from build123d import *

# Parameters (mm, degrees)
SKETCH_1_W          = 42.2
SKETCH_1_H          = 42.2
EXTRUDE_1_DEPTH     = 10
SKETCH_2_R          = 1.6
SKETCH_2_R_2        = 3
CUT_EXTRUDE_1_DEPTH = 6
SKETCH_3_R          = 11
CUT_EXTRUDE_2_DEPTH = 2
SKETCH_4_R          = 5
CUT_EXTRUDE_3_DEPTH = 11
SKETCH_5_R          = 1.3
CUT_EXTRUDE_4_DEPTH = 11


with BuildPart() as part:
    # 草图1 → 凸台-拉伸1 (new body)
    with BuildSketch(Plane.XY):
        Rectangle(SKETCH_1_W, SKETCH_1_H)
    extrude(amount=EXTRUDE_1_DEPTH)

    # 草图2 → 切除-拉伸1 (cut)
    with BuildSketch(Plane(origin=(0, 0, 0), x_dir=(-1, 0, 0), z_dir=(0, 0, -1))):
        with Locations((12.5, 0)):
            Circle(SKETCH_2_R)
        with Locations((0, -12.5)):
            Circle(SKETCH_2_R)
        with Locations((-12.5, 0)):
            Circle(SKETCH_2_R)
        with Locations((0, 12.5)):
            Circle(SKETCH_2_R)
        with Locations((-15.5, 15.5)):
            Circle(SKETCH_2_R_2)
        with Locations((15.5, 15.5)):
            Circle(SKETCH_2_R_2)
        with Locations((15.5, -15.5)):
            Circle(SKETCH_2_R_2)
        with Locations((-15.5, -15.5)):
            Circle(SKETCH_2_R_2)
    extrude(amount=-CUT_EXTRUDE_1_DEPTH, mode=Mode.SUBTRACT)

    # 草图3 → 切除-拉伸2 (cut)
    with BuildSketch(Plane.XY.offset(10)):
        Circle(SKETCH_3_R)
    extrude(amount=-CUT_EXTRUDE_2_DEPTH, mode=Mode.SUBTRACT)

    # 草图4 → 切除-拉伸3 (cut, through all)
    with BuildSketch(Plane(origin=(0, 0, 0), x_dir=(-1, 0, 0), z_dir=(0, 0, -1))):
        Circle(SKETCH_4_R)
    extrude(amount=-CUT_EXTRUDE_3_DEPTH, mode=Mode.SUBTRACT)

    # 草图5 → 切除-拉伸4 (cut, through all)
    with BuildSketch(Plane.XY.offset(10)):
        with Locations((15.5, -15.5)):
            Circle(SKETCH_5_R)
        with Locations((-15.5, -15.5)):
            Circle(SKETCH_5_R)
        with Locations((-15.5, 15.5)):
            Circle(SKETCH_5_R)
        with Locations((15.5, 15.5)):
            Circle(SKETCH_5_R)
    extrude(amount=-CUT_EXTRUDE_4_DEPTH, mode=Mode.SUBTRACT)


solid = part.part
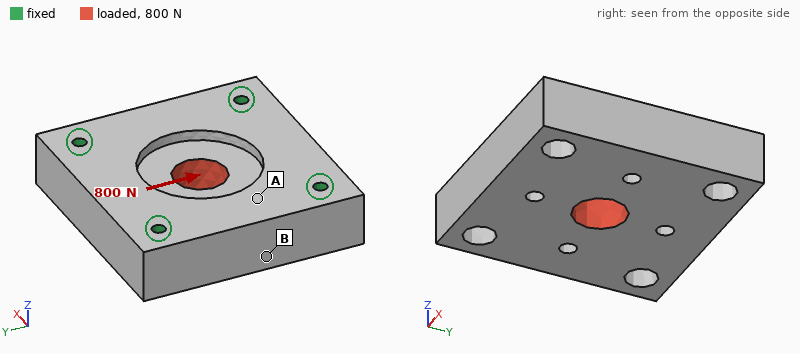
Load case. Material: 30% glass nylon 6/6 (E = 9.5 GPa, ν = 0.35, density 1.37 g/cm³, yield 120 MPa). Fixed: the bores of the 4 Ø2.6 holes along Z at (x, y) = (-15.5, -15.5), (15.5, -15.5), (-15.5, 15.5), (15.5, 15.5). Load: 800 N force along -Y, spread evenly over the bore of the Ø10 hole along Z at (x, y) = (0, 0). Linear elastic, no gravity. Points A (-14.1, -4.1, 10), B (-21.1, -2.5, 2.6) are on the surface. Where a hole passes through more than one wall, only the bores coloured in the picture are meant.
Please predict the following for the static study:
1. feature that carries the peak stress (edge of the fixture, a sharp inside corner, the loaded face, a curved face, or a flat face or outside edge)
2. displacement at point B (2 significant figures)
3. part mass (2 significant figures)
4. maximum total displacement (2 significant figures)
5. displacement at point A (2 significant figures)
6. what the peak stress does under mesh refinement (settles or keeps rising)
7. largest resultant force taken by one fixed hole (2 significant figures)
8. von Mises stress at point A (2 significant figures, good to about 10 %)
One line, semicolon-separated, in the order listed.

edge of the fixture; 2.8 µm; 21 g; 9.7 µm; 3.4 µm; keeps rising; 210 N; 1.6 MPa
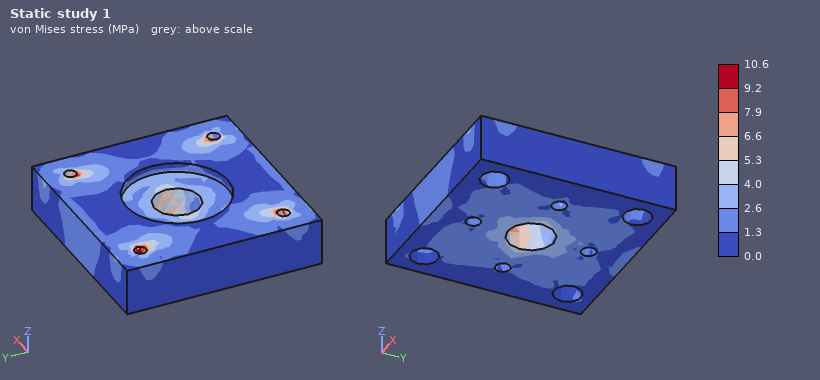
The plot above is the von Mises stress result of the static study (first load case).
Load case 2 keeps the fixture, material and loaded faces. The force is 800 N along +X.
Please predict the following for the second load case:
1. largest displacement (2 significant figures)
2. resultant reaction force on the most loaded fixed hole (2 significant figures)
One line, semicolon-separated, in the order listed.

9.8 µm; 220 N
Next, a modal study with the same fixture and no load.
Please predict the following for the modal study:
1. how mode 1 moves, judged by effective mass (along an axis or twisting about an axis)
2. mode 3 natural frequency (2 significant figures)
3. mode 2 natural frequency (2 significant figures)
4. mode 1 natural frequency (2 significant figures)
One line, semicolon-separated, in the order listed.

along Z; 14 kHz; 14 kHz; 10 kHz
